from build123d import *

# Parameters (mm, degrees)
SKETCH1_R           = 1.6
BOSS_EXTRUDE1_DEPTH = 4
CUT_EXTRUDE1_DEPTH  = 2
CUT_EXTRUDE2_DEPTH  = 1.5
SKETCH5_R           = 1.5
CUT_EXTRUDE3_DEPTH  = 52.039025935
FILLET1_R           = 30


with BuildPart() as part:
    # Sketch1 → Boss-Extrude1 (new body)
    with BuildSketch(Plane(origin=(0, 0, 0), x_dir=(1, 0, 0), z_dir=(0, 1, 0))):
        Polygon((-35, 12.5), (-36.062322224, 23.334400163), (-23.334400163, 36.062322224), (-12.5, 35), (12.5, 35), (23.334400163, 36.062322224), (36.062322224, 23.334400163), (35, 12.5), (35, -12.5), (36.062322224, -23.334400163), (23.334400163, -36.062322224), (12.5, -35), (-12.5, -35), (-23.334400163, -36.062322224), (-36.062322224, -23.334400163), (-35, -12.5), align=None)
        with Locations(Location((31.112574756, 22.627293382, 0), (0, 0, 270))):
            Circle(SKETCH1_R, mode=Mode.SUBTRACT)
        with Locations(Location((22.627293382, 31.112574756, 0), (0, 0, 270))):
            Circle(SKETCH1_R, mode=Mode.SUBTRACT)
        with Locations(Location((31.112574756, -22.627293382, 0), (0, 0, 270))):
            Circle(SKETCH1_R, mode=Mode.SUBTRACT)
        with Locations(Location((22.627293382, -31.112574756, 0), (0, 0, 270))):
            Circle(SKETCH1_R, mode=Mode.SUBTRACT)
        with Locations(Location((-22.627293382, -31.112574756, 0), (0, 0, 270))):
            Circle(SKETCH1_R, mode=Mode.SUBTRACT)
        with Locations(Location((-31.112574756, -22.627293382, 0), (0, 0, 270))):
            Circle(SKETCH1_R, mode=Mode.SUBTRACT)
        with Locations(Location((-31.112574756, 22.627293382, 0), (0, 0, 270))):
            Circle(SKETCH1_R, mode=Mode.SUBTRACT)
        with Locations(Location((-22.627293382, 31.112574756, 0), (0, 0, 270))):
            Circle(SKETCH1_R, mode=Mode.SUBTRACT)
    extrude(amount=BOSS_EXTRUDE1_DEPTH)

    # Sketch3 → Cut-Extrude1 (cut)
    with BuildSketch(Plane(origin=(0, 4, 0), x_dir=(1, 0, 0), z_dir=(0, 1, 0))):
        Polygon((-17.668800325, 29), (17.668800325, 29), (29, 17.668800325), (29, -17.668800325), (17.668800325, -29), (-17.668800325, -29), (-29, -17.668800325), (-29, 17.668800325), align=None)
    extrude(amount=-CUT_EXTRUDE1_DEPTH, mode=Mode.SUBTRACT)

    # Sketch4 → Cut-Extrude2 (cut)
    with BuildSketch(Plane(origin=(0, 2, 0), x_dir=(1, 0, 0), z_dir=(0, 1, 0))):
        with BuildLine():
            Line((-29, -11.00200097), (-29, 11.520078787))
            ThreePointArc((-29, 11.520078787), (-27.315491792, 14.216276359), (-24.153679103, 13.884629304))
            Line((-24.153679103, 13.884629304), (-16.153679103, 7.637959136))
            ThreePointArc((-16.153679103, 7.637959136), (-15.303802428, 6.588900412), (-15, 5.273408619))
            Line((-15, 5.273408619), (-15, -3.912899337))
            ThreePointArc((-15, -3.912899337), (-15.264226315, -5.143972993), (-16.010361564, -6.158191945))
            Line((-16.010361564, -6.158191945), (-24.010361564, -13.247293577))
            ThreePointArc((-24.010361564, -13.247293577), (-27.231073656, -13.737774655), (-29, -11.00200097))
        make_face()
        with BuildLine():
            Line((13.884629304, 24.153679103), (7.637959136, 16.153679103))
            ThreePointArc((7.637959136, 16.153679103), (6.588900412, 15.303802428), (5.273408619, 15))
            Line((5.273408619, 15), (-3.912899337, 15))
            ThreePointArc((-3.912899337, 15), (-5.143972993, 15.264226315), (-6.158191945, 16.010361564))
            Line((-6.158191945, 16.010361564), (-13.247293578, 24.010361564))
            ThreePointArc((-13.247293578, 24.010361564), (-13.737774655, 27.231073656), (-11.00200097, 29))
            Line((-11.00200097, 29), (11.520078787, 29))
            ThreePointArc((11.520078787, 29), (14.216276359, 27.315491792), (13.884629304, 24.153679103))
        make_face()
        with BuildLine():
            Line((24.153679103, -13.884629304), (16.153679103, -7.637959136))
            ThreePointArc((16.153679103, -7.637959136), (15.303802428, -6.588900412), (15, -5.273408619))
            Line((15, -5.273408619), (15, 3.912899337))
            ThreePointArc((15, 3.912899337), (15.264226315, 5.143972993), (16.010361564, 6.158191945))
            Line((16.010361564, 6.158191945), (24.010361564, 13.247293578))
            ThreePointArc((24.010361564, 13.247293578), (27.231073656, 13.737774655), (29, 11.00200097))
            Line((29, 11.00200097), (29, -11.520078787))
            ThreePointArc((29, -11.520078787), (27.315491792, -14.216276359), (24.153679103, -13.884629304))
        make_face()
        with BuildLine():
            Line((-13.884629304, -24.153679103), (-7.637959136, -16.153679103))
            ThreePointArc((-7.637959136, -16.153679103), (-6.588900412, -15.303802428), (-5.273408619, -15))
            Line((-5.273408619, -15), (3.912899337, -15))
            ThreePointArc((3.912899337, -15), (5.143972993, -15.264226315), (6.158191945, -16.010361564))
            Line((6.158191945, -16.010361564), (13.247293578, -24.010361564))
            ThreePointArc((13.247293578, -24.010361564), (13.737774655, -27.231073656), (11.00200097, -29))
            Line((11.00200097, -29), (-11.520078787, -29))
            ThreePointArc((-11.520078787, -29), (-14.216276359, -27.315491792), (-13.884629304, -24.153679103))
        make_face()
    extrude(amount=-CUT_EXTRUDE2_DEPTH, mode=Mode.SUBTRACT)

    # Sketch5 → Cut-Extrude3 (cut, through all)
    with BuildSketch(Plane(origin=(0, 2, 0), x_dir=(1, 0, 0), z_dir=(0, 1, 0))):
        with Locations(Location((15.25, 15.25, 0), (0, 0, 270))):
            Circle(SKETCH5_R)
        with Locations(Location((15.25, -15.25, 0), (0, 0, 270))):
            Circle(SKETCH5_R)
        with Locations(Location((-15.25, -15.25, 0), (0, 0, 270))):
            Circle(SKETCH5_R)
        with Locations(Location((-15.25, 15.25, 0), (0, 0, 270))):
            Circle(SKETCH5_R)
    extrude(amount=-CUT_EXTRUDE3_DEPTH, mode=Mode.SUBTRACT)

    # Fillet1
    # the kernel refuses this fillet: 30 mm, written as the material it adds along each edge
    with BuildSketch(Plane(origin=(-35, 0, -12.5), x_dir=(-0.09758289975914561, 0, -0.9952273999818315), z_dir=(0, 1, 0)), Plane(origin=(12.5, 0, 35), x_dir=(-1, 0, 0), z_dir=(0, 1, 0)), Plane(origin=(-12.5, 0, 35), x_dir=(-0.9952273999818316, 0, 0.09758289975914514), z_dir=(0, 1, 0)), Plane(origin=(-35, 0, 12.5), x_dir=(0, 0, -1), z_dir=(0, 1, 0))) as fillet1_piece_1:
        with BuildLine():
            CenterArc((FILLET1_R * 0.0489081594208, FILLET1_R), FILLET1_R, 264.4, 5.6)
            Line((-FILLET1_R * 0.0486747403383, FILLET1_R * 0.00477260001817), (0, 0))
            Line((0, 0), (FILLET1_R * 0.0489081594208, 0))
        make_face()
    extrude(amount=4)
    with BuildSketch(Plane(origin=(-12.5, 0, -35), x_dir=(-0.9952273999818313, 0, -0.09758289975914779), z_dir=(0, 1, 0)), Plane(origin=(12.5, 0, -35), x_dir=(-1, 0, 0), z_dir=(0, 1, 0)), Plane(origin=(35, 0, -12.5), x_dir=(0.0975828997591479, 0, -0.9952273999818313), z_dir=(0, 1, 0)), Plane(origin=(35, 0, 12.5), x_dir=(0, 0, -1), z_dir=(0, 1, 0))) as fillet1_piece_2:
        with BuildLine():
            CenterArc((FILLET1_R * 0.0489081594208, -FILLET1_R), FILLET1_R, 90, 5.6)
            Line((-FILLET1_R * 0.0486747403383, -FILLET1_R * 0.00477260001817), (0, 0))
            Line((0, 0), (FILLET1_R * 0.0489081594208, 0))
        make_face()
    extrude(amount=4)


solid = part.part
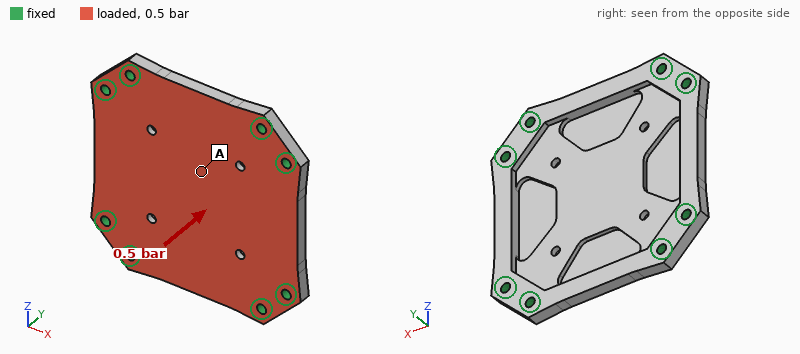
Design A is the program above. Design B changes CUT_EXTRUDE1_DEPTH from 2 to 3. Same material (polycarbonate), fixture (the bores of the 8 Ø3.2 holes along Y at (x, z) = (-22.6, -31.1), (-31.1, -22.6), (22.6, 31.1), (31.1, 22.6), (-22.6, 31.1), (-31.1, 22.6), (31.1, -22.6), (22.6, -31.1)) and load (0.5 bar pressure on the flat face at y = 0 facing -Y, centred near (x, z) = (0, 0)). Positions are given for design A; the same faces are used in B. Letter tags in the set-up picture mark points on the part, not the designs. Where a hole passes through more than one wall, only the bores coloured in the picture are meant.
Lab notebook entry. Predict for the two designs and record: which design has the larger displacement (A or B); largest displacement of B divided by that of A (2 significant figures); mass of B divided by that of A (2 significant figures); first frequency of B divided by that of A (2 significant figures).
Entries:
B
5.5
0.83
0.59
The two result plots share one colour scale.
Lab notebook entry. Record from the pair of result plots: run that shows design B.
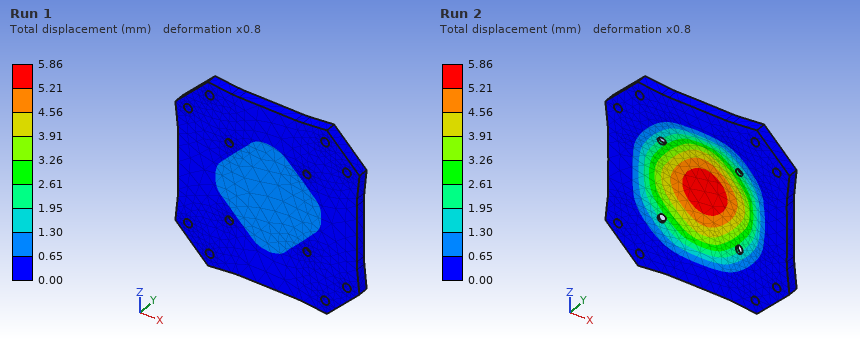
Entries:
Run 2
